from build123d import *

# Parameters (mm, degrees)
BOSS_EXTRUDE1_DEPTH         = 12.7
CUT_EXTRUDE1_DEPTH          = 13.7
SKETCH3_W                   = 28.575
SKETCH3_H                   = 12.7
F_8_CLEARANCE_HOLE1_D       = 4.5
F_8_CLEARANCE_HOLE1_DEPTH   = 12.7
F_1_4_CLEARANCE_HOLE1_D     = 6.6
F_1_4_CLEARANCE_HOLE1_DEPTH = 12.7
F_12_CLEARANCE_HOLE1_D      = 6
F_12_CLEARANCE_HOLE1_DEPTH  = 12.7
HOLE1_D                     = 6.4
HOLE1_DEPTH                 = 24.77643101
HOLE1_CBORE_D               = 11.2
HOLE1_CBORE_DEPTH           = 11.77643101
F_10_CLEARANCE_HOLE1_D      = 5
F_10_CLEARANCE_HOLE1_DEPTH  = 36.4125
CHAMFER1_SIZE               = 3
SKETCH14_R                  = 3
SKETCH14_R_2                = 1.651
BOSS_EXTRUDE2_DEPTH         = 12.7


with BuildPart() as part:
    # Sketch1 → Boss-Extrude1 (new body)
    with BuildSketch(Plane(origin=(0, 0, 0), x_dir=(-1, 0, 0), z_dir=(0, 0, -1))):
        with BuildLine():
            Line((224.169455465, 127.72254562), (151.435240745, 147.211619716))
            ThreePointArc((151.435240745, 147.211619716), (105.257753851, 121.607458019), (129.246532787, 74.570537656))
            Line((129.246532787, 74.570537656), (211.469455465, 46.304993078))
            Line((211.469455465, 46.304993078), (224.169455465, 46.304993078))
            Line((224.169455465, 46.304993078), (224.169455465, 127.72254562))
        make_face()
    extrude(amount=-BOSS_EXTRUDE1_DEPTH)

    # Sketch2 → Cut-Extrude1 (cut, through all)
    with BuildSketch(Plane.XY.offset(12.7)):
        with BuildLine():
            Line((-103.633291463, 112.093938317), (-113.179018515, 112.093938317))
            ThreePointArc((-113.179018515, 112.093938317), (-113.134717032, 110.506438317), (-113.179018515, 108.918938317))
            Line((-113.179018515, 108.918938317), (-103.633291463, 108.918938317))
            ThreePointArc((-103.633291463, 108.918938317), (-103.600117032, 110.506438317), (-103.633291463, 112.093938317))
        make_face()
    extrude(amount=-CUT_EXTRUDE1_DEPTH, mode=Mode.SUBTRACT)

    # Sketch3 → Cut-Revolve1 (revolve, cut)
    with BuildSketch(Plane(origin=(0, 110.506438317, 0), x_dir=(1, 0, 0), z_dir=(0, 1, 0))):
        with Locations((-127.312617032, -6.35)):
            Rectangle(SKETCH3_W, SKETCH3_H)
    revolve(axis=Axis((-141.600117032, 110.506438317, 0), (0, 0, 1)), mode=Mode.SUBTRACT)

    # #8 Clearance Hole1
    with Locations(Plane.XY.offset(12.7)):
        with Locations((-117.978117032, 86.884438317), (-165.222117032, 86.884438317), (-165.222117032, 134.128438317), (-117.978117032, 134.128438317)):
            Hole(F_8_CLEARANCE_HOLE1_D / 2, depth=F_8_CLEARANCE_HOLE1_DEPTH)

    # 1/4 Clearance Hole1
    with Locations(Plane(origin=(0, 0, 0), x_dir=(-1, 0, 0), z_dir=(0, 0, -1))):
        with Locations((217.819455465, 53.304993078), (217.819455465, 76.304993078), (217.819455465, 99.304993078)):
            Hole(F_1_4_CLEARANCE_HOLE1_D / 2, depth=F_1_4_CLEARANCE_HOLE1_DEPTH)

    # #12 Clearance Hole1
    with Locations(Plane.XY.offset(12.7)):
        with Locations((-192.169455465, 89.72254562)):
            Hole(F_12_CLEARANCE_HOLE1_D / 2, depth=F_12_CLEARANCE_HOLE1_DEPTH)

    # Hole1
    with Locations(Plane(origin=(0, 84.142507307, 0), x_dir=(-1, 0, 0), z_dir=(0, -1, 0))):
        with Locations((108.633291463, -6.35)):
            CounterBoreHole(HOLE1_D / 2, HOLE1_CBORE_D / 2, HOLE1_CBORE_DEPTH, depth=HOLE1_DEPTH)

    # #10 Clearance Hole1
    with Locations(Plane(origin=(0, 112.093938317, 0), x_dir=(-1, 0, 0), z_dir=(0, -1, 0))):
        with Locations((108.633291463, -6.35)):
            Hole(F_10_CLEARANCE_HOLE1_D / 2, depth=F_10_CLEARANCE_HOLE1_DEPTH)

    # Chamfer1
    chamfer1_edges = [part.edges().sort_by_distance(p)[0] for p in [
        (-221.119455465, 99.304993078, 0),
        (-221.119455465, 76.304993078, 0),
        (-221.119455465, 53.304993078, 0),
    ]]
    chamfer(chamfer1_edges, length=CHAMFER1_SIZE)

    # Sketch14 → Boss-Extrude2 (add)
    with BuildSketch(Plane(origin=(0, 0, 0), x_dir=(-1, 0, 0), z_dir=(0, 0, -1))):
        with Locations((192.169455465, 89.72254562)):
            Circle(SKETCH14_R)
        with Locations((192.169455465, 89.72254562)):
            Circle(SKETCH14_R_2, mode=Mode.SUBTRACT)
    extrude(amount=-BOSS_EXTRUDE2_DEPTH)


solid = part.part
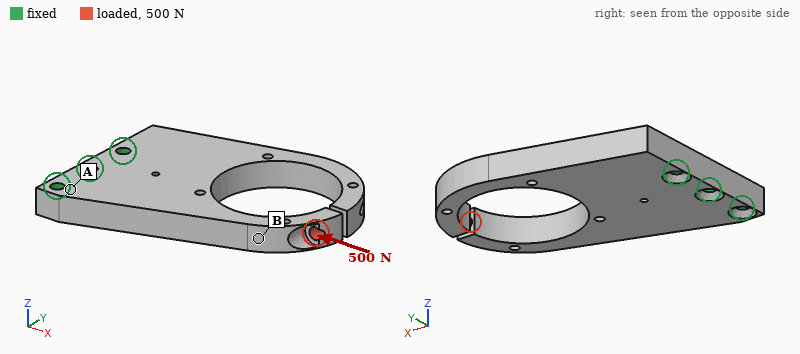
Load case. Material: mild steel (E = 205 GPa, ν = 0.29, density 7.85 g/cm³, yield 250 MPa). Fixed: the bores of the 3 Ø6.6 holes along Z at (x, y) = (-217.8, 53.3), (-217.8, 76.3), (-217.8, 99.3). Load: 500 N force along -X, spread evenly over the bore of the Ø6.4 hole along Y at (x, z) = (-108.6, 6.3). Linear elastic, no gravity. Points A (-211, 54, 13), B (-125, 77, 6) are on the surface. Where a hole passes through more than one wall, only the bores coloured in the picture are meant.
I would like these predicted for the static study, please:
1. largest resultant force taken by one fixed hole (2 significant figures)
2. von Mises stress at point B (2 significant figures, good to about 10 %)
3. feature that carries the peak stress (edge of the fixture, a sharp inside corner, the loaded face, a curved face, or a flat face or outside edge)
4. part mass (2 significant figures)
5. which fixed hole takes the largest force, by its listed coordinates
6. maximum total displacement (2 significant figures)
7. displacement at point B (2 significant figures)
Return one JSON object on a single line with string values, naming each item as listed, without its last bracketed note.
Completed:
{"largest resultant force taken by one fixed hole": "460 N", "von Mises stress at point B": "50 MPa", "feature that carries the peak stress": "a curved face", "part mass": "620 g", "which fixed hole takes the largest force, by its listed coordinates": "(-217.8, 99.3)", "maximum total displacement": "0.10 mm", "displacement at point B": "0.019 mm"}
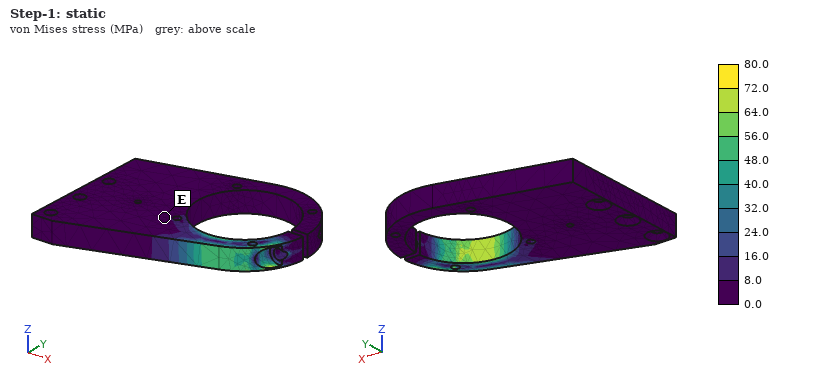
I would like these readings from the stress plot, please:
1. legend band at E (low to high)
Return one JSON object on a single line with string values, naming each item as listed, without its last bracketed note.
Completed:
{"legend band at E": "0.0 to 8.0 MPa"}
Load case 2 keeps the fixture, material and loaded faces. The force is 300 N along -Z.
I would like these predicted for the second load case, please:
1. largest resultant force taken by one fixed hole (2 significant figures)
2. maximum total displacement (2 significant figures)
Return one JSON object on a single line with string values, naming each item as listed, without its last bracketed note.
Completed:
{"largest resultant force taken by one fixed hole": "220 N", "maximum total displacement": "0.15 mm"}
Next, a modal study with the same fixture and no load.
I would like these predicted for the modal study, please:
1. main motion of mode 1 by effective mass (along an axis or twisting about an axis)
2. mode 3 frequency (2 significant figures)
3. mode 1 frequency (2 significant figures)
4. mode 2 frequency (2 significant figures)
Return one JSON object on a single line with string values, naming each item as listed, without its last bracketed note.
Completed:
{"main motion of mode 1 by effective mass": "along Z", "mode 3 frequency": "1600 Hz", "mode 1 frequency": "1000 Hz", "mode 2 frequency": "1600 Hz"}
